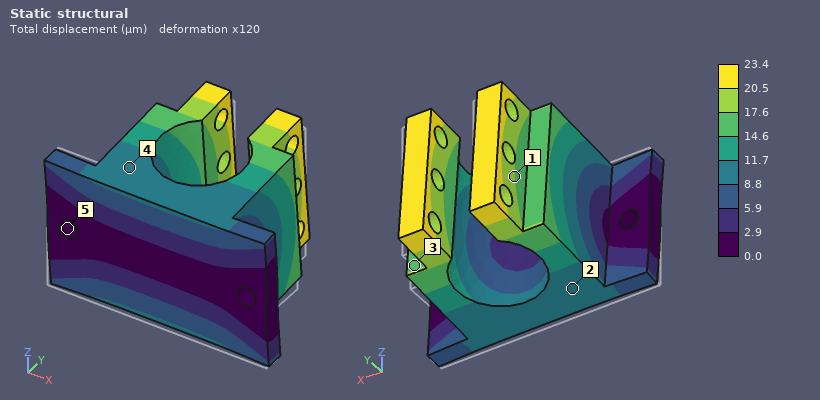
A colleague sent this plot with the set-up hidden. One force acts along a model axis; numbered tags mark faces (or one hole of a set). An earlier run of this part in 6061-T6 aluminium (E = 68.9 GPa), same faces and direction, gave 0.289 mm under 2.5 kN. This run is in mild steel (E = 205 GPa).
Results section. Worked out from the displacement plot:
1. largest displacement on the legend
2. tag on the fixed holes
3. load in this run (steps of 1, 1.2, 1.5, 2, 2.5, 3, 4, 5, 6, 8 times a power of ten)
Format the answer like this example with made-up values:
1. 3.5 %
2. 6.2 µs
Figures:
1. 23.4 µm
2. 5
3. 600 N
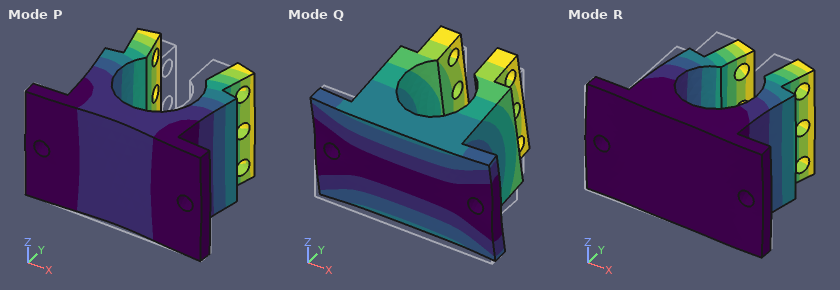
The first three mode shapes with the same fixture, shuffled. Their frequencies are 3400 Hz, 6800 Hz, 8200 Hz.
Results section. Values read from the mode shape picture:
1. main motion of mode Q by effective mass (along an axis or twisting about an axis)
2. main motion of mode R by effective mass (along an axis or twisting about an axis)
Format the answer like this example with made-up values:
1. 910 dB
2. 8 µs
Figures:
1. along Z
2. along X
